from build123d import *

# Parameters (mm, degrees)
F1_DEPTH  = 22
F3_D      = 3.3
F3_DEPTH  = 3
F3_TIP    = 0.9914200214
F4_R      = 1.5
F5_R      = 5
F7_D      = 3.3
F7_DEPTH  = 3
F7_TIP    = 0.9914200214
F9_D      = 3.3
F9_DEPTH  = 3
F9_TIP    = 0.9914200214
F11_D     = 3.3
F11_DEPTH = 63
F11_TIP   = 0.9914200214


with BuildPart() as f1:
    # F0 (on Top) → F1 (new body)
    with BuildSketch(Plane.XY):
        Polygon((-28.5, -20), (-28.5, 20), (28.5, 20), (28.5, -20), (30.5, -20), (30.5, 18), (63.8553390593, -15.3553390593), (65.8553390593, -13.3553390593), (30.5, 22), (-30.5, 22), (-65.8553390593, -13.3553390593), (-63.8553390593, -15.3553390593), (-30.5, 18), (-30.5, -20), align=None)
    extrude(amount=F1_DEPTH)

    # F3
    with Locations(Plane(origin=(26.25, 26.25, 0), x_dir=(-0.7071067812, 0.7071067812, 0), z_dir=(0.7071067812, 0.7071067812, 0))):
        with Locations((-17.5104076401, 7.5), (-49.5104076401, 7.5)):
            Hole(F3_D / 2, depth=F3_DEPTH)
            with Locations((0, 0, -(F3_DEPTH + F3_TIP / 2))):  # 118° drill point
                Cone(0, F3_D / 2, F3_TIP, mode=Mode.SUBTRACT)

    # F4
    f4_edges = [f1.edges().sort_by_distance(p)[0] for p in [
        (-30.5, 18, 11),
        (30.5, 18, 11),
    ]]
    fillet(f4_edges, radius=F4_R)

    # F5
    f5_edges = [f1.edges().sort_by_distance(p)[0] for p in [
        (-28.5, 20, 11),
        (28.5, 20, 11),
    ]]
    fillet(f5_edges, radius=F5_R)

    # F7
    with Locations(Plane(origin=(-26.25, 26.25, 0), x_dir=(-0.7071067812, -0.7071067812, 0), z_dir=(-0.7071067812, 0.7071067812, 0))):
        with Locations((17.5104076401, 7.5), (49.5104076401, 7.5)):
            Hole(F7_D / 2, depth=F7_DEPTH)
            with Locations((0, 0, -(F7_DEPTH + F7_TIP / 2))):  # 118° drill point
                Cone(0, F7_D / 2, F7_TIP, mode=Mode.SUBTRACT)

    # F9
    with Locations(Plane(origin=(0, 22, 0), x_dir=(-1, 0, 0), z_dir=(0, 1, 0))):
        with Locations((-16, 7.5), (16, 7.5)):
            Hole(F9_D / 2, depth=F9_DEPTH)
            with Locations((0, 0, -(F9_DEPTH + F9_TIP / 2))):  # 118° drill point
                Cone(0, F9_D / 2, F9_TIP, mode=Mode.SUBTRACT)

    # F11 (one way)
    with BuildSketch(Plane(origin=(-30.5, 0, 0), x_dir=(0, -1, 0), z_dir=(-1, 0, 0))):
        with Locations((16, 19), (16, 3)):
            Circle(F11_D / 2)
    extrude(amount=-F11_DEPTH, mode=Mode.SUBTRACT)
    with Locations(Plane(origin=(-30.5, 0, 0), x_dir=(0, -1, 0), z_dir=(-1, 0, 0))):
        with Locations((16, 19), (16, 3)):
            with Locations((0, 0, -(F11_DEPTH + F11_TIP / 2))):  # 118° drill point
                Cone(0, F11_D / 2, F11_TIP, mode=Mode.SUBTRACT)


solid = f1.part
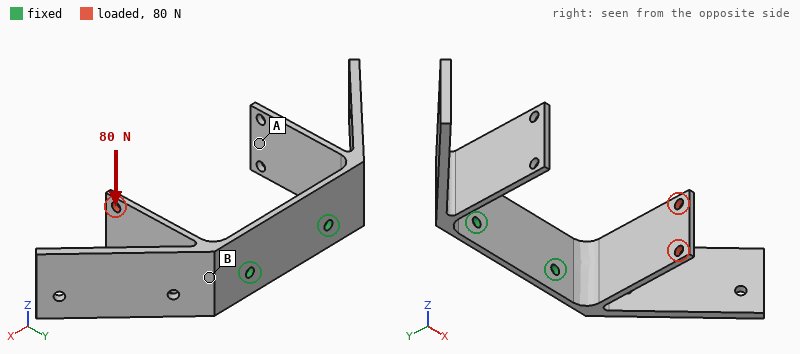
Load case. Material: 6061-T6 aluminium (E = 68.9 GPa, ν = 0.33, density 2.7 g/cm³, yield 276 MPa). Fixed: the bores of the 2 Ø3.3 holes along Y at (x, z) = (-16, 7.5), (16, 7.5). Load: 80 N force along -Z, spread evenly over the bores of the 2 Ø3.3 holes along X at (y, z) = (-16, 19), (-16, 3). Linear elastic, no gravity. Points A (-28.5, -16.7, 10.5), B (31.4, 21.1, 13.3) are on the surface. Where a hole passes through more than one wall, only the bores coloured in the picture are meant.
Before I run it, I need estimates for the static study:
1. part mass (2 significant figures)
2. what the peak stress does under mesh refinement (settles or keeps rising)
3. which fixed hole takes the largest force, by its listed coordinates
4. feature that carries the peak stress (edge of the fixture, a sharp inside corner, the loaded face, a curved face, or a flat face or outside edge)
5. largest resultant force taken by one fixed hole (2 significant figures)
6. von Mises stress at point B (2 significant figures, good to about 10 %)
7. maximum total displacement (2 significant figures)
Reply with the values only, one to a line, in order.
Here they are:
34 g
keeps rising
(16, 7.5)
edge of the fixture
110 N
28 MPa
0.67 mm
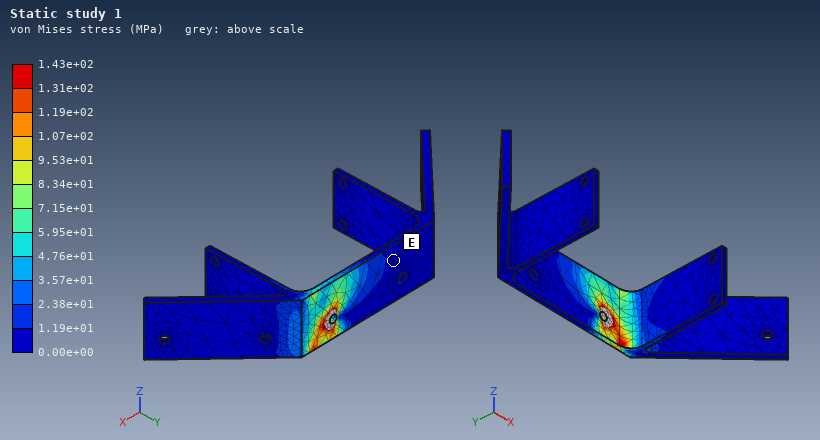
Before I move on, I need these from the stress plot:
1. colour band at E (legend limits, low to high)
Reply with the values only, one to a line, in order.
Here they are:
0.00e+00 to 1.19e+01 MPa
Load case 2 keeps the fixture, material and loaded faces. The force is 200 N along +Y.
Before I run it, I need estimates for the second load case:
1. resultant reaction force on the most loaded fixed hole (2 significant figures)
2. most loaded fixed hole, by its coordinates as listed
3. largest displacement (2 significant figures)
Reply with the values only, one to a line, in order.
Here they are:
220 N
(16, 7.5)
1.0 mm
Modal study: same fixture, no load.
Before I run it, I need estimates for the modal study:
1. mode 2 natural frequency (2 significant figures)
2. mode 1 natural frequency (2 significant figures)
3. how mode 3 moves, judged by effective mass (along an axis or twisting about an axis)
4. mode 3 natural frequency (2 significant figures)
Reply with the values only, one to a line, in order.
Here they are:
410 Hz
410 Hz
along Z
860 Hz
